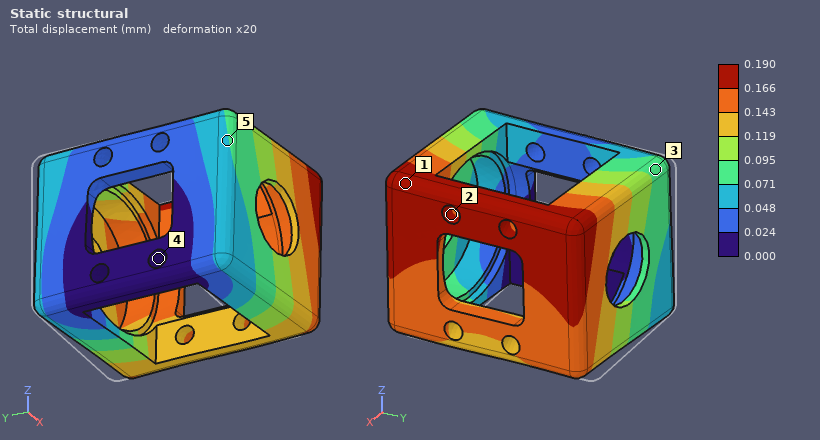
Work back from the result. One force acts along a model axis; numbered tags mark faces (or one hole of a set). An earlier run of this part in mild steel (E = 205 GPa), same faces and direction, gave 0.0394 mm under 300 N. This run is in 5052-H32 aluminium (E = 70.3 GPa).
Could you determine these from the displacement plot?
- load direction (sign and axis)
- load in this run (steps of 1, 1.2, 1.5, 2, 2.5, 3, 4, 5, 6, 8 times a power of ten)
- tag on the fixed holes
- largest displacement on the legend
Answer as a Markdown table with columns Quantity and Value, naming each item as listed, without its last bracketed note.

| Quantity | Value |
|---|---|
| load direction | -Y |
| load in this run | 500 N |
| tag on the fixed holes | 4 |
| largest displacement on the legend | 0.190 mm |
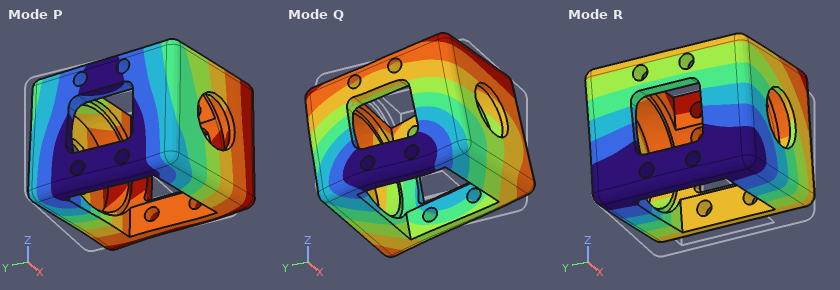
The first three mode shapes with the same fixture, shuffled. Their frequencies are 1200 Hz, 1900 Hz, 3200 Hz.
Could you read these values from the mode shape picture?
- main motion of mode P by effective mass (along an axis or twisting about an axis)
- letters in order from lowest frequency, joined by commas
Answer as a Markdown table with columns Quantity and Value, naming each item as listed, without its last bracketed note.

| Quantity | Value |
|---|---|
| main motion of mode P by effective mass | along Y |
| letters in order from lowest frequency, joined by commas | R, P, Q |
